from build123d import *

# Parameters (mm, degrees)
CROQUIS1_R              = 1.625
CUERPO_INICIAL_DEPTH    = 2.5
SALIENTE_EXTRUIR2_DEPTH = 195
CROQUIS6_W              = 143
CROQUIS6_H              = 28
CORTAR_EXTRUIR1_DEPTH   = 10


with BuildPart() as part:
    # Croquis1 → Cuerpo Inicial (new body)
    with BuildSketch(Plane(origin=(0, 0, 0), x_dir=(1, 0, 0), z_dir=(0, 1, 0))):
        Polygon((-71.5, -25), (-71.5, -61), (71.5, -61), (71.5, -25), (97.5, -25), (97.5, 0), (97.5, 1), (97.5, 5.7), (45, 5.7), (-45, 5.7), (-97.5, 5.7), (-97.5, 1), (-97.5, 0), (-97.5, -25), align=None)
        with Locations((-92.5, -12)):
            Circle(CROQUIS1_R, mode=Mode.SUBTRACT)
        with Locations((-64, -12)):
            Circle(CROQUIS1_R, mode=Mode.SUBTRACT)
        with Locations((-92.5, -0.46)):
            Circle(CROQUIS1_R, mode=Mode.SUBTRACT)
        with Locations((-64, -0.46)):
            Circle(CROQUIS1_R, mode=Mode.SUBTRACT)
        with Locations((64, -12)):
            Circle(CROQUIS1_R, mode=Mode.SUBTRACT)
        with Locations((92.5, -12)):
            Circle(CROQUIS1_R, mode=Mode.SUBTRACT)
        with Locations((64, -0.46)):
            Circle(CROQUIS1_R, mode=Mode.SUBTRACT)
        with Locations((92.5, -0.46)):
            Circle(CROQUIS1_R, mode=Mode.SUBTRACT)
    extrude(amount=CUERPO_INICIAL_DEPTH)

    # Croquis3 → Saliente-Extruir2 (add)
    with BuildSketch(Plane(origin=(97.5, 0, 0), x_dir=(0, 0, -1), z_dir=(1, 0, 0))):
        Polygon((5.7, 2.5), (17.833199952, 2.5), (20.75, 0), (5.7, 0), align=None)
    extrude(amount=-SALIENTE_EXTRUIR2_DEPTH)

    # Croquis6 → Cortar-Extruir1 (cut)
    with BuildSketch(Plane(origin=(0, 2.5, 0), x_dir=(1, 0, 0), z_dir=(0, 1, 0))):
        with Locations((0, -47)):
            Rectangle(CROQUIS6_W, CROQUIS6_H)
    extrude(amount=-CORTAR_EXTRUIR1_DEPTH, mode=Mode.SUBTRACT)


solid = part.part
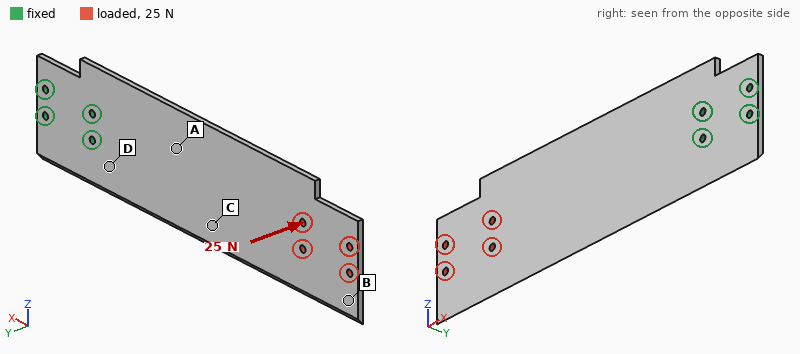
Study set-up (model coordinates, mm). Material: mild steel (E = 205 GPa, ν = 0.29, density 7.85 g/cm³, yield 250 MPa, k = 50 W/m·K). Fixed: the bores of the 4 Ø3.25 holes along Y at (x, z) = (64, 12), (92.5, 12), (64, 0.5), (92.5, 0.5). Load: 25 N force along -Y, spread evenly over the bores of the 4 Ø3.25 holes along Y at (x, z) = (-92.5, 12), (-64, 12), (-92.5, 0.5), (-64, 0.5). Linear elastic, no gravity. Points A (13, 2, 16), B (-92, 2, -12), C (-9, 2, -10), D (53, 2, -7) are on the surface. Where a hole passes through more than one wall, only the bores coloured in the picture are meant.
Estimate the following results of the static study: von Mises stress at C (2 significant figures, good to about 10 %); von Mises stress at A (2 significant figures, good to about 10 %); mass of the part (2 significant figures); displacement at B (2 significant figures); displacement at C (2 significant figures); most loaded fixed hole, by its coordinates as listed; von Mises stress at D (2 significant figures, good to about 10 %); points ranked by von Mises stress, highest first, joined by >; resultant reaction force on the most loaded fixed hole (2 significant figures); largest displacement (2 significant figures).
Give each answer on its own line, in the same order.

33 MPa
41 MPa
190 g
2.0 mm
0.57 mm
(64, 0.5)
60 MPa
D > A > C > B
37 N
2.1 mm
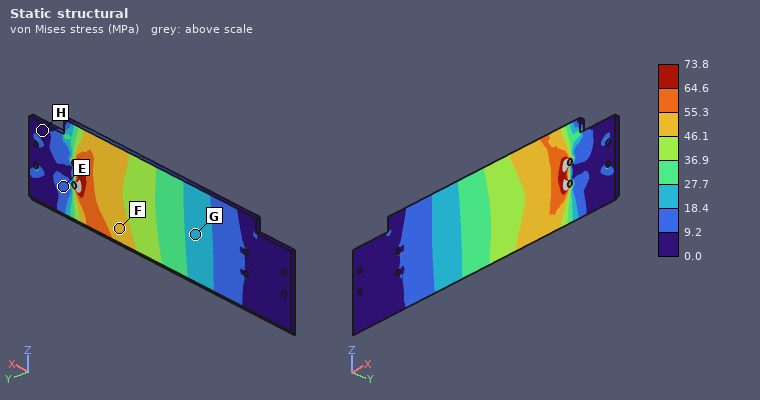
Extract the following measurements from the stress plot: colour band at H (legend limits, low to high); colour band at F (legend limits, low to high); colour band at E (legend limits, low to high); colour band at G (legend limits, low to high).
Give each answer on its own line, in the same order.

0.0 to 9.2 MPa
46.1 to 55.3 MPa
9.2 to 18.4 MPa
18.4 to 27.7 MPa
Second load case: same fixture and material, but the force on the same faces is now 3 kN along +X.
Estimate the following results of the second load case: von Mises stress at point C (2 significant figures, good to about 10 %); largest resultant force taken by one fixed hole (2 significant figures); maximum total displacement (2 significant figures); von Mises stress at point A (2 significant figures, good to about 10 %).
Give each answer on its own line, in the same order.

25 MPa
1.3 kN
35 µm
23 MPa
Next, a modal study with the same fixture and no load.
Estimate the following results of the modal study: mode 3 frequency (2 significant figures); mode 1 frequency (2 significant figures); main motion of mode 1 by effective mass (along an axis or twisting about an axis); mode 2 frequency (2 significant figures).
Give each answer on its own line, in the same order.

530 Hz
82 Hz
along Y
490 Hz
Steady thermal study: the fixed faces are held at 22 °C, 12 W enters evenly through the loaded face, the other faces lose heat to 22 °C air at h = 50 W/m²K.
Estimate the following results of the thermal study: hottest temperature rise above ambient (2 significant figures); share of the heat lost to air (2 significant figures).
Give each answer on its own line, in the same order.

52 K
98 %
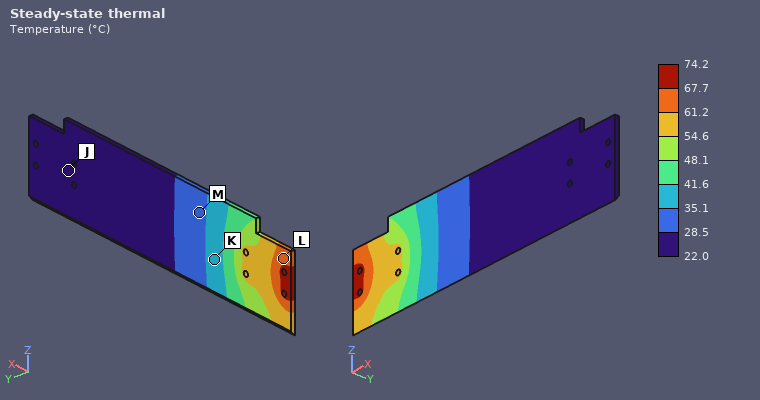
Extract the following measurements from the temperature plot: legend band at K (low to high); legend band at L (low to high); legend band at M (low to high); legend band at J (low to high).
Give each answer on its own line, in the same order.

35.1 to 41.6 °C
61.2 to 67.7 °C
28.5 to 35.1 °C
22.0 to 28.5 °C
